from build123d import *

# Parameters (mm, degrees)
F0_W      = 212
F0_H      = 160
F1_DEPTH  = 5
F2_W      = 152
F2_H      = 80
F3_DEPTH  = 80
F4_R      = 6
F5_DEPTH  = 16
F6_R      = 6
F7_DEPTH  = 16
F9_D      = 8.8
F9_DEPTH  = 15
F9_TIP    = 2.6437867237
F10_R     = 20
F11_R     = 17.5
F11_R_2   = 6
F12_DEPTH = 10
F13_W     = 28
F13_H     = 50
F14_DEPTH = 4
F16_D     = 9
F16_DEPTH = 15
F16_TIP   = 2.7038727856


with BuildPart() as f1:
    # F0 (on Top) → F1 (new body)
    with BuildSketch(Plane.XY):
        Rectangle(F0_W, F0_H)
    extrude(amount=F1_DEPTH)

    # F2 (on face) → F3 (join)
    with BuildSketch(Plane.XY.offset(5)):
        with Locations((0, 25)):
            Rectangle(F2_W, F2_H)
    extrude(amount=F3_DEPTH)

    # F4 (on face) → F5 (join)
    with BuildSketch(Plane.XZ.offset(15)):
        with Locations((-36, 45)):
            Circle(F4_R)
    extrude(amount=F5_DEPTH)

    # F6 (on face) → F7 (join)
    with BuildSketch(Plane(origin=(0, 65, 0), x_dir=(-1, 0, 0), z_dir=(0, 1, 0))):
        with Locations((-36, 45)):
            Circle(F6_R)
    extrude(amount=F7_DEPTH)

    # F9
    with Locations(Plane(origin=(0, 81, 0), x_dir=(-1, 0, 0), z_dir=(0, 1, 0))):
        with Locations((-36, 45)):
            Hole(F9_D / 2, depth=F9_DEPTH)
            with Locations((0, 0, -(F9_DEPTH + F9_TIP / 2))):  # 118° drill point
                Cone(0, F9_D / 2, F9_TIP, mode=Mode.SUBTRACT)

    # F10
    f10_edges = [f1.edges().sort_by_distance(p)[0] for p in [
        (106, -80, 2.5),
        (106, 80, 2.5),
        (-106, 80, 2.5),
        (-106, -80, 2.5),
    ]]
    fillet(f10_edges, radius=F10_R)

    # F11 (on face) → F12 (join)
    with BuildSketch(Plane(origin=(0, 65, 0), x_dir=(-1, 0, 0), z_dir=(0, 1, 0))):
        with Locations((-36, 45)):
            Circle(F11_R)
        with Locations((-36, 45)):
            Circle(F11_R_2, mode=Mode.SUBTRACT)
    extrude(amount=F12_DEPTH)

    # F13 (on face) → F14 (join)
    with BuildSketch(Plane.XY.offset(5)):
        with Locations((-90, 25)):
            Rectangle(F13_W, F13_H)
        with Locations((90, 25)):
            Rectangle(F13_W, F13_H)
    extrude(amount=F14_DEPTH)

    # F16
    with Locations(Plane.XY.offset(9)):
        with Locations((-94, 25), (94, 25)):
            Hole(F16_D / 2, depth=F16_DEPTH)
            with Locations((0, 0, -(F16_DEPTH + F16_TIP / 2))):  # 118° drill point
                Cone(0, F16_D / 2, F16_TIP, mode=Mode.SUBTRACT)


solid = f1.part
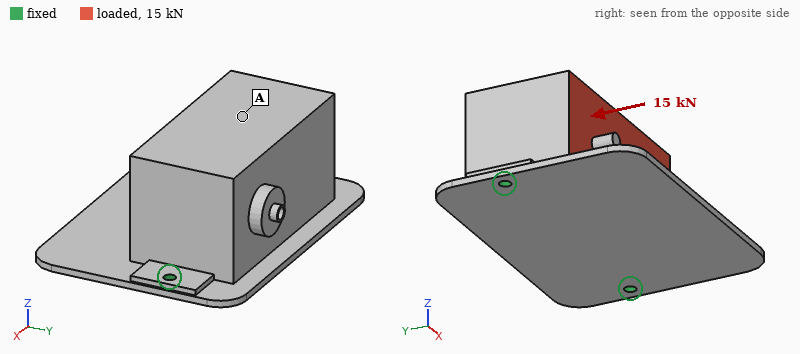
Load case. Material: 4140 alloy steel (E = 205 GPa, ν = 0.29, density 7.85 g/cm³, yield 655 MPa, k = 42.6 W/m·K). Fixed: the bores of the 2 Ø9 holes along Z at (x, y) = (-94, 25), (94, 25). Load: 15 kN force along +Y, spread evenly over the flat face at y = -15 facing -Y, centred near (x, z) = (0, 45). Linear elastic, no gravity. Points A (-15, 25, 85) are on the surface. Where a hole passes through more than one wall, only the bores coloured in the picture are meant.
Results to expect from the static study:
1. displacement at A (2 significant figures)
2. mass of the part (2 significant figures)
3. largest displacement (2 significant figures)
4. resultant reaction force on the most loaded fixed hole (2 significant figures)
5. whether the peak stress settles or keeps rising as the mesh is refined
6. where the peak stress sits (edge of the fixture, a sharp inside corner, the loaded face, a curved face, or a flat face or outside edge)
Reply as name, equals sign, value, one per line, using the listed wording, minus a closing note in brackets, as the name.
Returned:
displacement at A = 0.43 mm
mass of the part = 9.1 kg
largest displacement = 0.57 mm
resultant reaction force on the most loaded fixed hole = 7.5 kN
whether the peak stress settles or keeps rising as the mesh is refined = keeps rising
where the peak stress sits = edge of the fixture
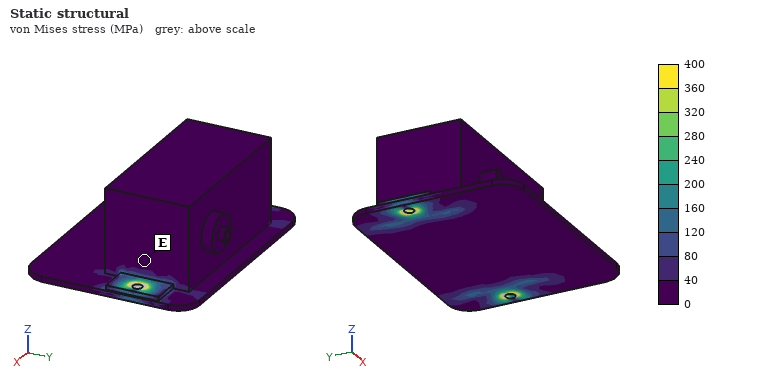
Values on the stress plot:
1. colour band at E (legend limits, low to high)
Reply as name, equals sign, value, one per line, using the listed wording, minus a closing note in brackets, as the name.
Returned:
colour band at E = 0 to 40 MPa
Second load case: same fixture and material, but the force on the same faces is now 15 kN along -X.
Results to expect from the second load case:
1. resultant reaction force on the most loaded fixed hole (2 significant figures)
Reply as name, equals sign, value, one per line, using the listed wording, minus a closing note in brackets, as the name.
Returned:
resultant reaction force on the most loaded fixed hole = 8.9 kN
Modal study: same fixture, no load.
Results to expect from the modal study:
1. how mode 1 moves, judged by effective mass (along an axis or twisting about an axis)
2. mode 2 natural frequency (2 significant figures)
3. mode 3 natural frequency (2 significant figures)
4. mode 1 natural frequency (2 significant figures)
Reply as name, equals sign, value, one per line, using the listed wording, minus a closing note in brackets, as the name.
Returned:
how mode 1 moves, judged by effective mass = along Y
mode 2 natural frequency = 970 Hz
mode 3 natural frequency = 1100 Hz
mode 1 natural frequency = 340 Hz
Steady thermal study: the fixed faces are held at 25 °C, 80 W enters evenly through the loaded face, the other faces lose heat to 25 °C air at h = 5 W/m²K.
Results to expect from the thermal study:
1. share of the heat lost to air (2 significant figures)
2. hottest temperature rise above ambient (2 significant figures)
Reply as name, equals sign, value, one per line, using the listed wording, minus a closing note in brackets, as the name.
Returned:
share of the heat lost to air = 25 %
hottest temperature rise above ambient = 53 K
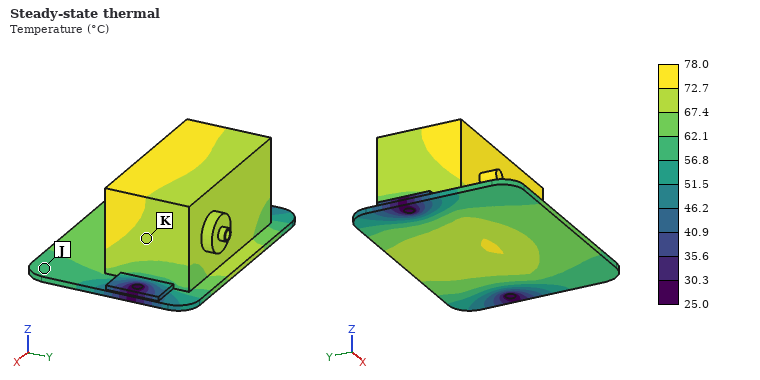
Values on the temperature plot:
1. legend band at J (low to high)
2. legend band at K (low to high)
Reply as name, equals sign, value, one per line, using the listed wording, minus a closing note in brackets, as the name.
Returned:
legend band at J = 56.8 to 62.1 °C
legend band at K = 67.4 to 72.7 °C
